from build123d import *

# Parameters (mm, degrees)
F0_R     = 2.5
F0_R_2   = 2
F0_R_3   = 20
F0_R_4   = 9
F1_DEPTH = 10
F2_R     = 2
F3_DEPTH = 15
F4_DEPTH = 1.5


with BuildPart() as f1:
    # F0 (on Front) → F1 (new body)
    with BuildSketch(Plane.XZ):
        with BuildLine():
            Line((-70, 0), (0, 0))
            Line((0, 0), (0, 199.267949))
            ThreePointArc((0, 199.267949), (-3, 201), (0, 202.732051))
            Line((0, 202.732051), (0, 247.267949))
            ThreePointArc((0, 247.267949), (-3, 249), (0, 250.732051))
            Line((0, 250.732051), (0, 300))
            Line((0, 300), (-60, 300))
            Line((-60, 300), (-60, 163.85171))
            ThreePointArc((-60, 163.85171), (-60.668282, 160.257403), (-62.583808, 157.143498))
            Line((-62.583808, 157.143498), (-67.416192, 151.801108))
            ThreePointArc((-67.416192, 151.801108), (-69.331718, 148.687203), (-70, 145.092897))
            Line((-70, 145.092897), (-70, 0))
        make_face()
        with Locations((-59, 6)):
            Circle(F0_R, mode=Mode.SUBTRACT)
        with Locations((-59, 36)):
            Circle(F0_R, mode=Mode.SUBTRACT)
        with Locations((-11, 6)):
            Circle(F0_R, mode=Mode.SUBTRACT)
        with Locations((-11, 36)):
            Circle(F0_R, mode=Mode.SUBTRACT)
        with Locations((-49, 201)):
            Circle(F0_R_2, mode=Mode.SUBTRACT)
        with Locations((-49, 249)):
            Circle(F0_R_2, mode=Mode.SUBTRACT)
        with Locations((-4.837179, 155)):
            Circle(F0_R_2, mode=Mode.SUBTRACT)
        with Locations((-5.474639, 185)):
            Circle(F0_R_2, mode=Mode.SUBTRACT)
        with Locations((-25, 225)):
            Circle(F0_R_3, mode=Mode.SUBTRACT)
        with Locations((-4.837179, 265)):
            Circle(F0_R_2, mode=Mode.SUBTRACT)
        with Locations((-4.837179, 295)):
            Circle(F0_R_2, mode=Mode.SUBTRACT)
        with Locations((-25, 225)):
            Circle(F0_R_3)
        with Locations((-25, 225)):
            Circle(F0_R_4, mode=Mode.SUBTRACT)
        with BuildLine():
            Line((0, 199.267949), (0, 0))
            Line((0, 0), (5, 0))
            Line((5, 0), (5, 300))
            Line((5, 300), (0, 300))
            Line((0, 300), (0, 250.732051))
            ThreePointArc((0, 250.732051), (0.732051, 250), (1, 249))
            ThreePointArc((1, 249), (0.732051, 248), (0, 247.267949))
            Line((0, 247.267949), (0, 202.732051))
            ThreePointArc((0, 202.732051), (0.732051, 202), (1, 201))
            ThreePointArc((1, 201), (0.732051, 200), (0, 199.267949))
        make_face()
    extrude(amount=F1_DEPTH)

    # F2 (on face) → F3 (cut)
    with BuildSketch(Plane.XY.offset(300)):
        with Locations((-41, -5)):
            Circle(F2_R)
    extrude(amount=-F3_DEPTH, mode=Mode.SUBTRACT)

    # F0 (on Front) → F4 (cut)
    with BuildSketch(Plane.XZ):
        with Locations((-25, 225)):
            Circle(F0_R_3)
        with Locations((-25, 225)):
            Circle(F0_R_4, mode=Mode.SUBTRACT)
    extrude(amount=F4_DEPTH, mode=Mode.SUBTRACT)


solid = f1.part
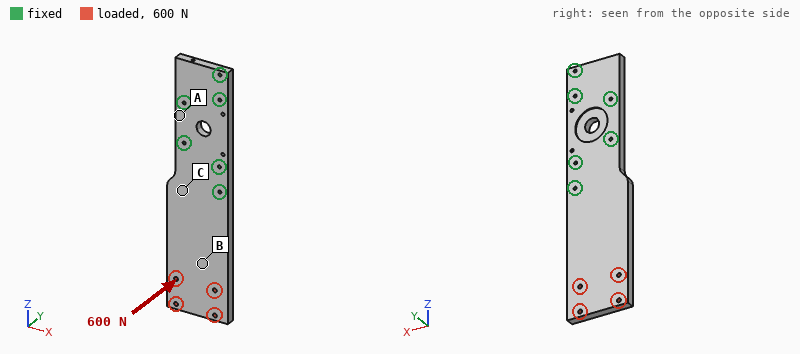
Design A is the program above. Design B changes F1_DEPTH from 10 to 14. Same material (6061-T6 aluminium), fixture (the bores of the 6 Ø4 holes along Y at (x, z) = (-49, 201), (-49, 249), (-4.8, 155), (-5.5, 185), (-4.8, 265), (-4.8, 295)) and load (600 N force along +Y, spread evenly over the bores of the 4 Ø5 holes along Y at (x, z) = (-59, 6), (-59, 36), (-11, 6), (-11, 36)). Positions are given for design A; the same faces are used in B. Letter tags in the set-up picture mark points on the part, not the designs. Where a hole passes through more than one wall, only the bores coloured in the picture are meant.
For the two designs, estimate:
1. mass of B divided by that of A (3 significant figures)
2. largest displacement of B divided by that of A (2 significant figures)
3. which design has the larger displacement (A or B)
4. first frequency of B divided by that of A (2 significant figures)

1.40
0.38
A
1.4
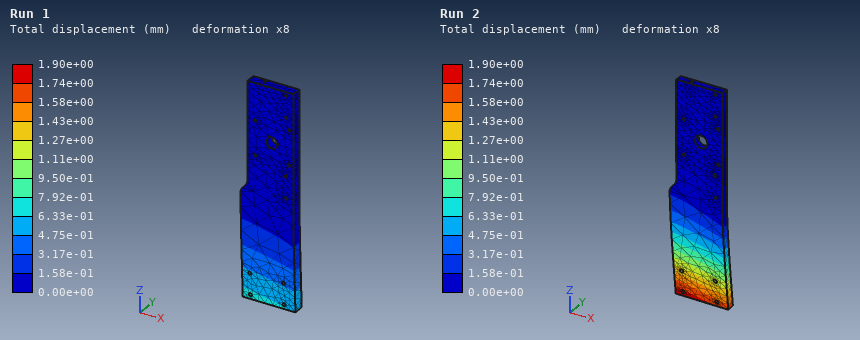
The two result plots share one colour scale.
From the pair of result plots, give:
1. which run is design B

Run 1
